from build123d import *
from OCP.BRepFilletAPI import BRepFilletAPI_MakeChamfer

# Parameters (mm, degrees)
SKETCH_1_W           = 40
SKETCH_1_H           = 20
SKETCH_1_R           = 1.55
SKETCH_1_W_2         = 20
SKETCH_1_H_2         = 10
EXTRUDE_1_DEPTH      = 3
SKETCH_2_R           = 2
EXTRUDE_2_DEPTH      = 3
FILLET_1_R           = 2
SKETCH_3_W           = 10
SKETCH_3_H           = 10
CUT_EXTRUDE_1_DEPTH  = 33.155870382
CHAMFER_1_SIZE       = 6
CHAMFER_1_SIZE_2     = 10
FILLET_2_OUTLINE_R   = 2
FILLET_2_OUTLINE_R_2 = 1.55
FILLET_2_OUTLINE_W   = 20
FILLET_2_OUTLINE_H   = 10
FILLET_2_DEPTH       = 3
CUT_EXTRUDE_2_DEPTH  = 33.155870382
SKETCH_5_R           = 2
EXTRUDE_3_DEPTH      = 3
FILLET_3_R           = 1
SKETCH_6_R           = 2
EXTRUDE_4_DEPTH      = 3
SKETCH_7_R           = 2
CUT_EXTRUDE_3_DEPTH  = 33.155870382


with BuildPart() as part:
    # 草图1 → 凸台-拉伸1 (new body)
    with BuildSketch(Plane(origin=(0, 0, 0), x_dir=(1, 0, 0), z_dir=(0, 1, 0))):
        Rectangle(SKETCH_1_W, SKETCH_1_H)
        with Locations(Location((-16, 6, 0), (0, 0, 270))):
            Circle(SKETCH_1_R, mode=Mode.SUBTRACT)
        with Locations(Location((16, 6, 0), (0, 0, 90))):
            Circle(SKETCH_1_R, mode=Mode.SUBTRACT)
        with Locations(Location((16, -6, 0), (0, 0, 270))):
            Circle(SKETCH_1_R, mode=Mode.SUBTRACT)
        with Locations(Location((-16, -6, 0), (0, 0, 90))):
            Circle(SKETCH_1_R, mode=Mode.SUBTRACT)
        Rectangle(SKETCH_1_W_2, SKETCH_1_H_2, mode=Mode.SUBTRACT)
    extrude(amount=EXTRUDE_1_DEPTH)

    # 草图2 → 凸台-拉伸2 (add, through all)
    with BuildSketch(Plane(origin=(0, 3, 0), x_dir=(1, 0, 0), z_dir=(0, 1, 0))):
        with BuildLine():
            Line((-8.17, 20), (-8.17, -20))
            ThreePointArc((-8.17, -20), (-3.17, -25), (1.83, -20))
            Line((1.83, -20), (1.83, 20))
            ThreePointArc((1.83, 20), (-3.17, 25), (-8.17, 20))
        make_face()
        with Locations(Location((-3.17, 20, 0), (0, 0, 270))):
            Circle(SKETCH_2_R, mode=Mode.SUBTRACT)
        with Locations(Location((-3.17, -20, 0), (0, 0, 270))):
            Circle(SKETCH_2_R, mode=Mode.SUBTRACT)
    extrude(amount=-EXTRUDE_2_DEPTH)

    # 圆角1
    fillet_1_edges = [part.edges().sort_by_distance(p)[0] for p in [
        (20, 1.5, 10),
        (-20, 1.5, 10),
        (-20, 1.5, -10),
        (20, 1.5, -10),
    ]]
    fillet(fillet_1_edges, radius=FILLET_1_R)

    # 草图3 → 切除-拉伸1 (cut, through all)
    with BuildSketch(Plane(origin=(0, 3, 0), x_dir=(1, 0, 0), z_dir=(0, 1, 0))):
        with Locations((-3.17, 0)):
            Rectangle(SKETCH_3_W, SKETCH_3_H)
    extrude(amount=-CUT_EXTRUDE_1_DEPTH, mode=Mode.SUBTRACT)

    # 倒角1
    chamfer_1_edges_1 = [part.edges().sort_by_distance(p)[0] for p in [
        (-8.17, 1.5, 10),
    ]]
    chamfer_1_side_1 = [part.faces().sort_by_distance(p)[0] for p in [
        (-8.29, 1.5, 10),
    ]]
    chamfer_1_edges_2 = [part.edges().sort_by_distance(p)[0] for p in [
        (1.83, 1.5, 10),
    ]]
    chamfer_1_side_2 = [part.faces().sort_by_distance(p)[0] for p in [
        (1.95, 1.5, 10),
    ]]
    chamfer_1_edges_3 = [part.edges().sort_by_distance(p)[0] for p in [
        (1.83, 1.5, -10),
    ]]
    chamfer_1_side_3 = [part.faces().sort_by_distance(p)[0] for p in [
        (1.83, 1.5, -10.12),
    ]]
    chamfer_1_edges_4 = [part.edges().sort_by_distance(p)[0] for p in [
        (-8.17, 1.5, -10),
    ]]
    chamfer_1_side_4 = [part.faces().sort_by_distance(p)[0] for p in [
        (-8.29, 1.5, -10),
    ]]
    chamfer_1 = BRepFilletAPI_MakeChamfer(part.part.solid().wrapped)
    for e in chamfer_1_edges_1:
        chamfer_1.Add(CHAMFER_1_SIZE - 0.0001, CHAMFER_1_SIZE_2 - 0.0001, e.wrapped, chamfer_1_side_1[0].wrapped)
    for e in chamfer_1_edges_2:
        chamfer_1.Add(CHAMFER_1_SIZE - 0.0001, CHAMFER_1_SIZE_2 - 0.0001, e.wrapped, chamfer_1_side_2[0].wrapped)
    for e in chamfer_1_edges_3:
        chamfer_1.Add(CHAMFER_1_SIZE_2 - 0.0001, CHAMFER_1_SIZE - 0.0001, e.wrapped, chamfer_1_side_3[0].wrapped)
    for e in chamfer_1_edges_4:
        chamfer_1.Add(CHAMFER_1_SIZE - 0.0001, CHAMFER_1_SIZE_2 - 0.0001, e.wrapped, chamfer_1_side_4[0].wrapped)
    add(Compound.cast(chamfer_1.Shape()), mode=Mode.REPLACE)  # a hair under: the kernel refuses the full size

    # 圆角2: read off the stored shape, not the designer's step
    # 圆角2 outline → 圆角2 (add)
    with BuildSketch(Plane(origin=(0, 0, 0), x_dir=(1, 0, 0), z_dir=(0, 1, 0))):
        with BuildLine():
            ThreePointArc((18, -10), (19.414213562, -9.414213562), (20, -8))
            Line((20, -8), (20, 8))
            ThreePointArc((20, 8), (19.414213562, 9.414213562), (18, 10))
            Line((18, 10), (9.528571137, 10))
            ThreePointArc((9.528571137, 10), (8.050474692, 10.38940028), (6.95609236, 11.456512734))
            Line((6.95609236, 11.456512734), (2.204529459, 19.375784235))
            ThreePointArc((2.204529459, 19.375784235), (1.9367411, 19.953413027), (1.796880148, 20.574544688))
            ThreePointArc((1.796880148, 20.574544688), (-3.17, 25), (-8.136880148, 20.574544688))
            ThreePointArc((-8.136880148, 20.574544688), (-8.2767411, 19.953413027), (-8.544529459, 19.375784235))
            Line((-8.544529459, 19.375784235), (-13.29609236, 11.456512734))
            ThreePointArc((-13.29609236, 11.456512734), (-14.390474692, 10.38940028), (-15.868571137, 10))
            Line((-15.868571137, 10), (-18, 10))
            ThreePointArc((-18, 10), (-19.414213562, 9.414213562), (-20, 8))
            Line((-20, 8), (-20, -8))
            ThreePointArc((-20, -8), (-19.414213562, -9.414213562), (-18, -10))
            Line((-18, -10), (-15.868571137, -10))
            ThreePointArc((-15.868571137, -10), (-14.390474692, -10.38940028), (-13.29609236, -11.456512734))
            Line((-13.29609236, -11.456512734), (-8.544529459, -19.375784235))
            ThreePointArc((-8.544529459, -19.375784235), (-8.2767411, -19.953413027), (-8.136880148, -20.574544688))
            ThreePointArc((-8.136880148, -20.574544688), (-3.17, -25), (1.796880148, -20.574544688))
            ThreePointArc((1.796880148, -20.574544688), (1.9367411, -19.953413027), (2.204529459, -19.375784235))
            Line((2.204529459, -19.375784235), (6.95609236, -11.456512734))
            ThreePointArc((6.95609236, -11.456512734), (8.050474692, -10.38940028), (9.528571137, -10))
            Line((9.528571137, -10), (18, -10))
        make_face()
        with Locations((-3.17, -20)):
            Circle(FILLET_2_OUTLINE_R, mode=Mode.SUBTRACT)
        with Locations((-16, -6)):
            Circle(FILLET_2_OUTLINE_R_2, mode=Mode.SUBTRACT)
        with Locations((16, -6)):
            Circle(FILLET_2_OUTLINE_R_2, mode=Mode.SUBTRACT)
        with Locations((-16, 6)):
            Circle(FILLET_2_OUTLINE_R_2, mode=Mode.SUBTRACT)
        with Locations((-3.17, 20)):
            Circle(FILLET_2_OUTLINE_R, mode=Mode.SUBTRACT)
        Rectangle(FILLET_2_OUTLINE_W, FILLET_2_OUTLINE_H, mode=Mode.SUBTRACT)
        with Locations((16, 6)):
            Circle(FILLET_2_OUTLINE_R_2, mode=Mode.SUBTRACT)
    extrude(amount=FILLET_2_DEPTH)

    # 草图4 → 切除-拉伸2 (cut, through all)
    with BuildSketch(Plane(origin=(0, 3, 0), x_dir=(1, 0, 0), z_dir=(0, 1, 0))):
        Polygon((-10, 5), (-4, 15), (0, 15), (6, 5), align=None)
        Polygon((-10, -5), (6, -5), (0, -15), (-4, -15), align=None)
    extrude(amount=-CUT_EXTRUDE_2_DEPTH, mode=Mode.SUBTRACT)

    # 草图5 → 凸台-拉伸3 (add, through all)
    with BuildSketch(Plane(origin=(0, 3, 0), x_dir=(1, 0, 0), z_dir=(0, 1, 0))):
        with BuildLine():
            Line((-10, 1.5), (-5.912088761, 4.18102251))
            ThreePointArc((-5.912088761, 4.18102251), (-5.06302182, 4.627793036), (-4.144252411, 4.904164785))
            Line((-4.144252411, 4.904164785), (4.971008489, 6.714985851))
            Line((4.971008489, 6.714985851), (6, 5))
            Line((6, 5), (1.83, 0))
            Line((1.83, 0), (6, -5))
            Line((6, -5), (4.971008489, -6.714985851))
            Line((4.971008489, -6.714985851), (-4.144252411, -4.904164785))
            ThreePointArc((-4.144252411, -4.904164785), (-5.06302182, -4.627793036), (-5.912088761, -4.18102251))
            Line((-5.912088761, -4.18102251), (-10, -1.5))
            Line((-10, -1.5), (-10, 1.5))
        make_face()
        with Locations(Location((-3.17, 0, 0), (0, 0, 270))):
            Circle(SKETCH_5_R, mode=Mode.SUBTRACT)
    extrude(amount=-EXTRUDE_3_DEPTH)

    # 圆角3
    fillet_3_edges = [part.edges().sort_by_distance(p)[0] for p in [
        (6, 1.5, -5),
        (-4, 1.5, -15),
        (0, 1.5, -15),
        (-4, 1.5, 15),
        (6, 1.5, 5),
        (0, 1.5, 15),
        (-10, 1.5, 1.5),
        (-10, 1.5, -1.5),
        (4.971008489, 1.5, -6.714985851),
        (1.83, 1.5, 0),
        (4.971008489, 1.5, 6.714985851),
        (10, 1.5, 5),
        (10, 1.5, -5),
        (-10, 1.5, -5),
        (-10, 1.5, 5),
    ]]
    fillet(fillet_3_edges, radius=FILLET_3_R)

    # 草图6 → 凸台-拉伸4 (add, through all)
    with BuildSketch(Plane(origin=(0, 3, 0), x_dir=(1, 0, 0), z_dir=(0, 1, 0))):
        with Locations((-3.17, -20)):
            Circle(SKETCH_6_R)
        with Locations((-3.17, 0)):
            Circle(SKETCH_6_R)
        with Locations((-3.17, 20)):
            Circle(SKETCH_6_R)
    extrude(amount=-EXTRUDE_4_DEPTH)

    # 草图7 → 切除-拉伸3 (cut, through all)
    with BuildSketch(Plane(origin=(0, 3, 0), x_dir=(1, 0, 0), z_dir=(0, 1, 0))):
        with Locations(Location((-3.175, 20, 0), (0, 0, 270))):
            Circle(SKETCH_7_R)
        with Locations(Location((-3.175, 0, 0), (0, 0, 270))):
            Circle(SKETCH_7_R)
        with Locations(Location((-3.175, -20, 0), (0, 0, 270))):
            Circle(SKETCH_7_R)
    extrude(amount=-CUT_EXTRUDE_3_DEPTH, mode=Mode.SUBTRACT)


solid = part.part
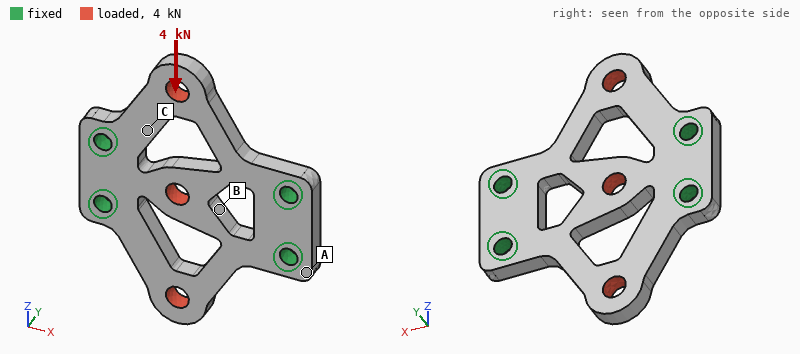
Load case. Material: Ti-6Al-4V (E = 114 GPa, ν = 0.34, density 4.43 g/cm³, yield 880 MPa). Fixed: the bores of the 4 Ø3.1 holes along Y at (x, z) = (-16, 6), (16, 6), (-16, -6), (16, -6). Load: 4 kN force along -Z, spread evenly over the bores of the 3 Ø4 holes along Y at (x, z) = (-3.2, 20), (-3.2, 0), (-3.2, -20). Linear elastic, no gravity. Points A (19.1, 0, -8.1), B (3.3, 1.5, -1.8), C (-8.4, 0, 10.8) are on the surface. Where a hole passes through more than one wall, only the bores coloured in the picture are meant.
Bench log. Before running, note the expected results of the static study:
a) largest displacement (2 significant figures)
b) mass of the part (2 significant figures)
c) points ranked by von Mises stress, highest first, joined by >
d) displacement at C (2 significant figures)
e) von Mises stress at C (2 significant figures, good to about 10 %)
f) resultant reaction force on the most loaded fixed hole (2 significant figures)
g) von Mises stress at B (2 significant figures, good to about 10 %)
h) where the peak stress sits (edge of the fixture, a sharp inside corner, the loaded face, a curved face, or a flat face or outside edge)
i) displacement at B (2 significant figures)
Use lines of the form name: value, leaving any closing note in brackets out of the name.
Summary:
largest displacement: 22 µm
mass of the part: 12 g
points ranked by von Mises stress, highest first, joined by >: B > C > A
displacement at C: 7.6 µm
von Mises stress at C: 56 MPa
resultant reaction force on the most loaded fixed hole: 1.2 kN
von Mises stress at B: 99 MPa
where the peak stress sits: a curved face
displacement at B: 22 µm
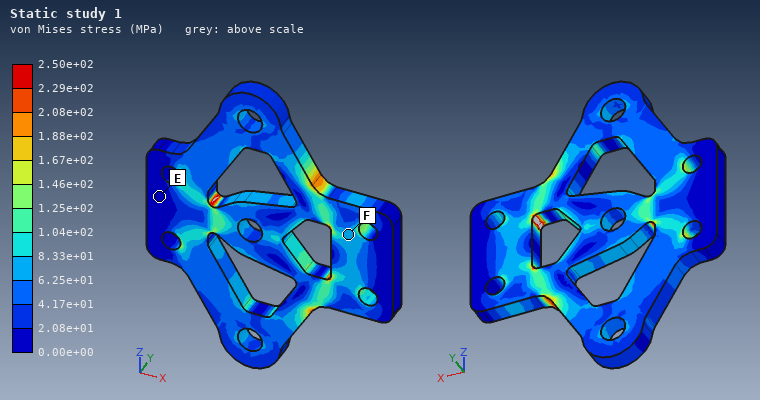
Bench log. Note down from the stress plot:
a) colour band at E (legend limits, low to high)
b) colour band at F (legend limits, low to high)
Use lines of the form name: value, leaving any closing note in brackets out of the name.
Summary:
colour band at E: 0.00e+00 to 2.08e+01 MPa
colour band at F: 6.25e+01 to 8.33e+01 MPa
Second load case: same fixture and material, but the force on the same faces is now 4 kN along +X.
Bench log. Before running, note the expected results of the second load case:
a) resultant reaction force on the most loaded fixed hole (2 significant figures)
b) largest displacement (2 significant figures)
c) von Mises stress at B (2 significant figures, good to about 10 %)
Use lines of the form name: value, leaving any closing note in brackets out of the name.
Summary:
resultant reaction force on the most loaded fixed hole: 1.2 kN
largest displacement: 25 µm
von Mises stress at B: 45 MPa
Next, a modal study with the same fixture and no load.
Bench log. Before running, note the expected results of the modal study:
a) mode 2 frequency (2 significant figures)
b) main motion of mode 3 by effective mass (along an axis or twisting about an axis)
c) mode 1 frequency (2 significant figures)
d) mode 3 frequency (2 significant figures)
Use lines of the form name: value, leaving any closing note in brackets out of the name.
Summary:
mode 2 frequency: 6400 Hz
main motion of mode 3 by effective mass: along Y
mode 1 frequency: 6300 Hz
mode 3 frequency: 16 kHz
